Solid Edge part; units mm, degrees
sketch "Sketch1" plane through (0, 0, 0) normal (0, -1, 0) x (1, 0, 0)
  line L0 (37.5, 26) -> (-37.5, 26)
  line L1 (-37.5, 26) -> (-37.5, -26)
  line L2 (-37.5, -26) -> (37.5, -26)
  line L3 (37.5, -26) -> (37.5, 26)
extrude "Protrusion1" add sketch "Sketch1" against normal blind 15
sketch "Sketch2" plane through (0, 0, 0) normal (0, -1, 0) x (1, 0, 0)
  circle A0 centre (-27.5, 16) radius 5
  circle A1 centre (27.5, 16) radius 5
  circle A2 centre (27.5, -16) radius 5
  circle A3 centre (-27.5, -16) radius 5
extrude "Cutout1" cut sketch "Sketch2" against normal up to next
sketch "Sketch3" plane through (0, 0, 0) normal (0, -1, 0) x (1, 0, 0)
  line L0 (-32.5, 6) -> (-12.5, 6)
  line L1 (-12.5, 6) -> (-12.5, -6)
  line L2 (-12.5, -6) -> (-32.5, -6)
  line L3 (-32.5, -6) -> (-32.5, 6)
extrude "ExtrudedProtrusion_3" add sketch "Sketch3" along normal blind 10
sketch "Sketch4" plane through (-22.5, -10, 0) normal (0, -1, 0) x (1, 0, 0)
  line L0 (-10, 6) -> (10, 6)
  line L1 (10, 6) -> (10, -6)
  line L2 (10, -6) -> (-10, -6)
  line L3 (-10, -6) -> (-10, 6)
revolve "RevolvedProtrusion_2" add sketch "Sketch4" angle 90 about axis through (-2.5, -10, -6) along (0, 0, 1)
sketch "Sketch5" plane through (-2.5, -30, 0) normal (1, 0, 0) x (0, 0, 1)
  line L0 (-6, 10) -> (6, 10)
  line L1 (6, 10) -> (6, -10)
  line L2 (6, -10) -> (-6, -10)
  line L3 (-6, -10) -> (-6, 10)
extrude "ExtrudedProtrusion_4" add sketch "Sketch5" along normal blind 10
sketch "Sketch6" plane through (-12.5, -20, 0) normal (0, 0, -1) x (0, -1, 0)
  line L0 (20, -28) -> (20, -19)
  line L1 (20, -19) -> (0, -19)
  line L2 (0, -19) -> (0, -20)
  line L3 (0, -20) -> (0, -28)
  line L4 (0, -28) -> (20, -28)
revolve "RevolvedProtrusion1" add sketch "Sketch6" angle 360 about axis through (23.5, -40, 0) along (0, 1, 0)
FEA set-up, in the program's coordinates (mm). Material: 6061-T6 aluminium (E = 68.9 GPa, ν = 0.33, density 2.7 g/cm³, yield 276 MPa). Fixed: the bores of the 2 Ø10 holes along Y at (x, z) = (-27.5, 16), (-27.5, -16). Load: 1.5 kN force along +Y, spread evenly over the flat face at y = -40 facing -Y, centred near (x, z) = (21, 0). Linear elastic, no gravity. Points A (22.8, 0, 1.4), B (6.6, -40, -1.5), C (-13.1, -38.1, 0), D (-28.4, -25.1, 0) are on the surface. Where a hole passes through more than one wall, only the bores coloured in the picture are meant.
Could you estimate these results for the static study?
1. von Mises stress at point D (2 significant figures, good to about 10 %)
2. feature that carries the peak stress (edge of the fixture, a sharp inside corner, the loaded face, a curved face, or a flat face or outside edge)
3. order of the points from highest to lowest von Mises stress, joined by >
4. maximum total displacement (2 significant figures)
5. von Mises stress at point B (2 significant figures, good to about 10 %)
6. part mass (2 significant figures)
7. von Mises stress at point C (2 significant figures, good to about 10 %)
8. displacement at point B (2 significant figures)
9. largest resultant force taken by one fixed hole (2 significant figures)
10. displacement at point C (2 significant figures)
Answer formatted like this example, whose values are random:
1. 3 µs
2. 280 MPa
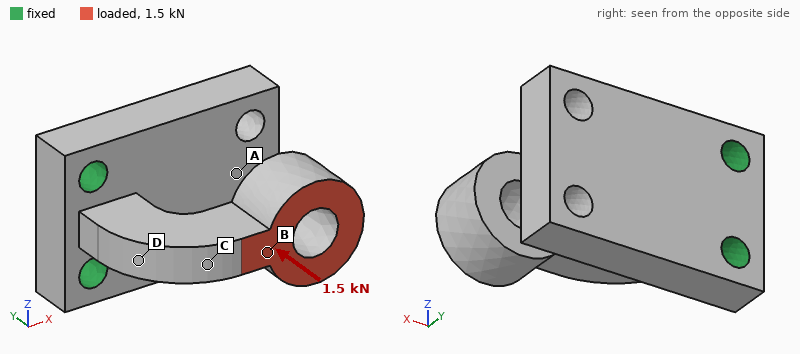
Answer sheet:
1. 51 MPa
2. a curved face
3. D > C > B > A
4. 0.37 mm
5. 22 MPa
6. 220 g
7. 40 MPa
8. 0.20 mm
9. 750 N
10. 0.13 mm
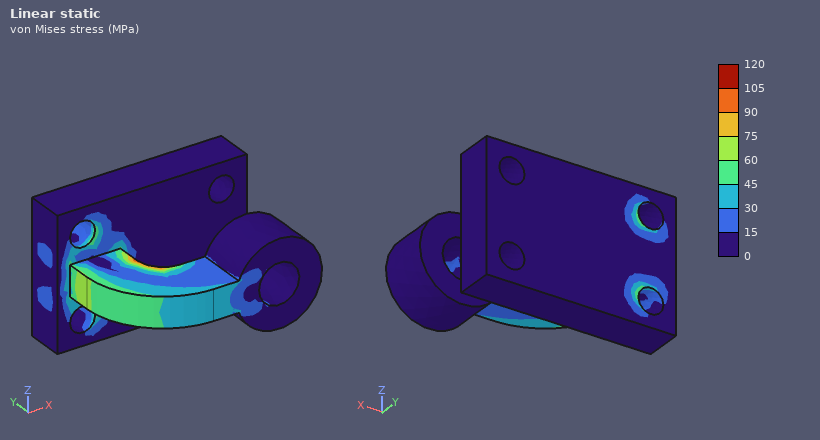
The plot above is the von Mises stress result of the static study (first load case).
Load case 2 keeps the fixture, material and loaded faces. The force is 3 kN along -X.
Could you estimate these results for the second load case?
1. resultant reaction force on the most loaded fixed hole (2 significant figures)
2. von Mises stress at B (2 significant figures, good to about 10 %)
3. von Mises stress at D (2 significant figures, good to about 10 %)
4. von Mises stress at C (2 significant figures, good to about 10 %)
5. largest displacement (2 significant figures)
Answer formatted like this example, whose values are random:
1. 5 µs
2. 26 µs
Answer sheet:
1. 1.7 kN
2. 31 MPa
3. 60 MPa
4. 42 MPa
5. 0.52 mm
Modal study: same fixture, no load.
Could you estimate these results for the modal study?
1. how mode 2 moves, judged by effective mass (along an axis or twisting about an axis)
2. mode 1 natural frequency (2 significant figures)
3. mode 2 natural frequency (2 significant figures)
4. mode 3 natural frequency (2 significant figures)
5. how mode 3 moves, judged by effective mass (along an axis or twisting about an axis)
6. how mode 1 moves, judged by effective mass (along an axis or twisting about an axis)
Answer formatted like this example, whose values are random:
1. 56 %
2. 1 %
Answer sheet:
1. along Y
2. 1100 Hz
3. 1700 Hz
4. 3300 Hz
5. along Y
6. along Z
